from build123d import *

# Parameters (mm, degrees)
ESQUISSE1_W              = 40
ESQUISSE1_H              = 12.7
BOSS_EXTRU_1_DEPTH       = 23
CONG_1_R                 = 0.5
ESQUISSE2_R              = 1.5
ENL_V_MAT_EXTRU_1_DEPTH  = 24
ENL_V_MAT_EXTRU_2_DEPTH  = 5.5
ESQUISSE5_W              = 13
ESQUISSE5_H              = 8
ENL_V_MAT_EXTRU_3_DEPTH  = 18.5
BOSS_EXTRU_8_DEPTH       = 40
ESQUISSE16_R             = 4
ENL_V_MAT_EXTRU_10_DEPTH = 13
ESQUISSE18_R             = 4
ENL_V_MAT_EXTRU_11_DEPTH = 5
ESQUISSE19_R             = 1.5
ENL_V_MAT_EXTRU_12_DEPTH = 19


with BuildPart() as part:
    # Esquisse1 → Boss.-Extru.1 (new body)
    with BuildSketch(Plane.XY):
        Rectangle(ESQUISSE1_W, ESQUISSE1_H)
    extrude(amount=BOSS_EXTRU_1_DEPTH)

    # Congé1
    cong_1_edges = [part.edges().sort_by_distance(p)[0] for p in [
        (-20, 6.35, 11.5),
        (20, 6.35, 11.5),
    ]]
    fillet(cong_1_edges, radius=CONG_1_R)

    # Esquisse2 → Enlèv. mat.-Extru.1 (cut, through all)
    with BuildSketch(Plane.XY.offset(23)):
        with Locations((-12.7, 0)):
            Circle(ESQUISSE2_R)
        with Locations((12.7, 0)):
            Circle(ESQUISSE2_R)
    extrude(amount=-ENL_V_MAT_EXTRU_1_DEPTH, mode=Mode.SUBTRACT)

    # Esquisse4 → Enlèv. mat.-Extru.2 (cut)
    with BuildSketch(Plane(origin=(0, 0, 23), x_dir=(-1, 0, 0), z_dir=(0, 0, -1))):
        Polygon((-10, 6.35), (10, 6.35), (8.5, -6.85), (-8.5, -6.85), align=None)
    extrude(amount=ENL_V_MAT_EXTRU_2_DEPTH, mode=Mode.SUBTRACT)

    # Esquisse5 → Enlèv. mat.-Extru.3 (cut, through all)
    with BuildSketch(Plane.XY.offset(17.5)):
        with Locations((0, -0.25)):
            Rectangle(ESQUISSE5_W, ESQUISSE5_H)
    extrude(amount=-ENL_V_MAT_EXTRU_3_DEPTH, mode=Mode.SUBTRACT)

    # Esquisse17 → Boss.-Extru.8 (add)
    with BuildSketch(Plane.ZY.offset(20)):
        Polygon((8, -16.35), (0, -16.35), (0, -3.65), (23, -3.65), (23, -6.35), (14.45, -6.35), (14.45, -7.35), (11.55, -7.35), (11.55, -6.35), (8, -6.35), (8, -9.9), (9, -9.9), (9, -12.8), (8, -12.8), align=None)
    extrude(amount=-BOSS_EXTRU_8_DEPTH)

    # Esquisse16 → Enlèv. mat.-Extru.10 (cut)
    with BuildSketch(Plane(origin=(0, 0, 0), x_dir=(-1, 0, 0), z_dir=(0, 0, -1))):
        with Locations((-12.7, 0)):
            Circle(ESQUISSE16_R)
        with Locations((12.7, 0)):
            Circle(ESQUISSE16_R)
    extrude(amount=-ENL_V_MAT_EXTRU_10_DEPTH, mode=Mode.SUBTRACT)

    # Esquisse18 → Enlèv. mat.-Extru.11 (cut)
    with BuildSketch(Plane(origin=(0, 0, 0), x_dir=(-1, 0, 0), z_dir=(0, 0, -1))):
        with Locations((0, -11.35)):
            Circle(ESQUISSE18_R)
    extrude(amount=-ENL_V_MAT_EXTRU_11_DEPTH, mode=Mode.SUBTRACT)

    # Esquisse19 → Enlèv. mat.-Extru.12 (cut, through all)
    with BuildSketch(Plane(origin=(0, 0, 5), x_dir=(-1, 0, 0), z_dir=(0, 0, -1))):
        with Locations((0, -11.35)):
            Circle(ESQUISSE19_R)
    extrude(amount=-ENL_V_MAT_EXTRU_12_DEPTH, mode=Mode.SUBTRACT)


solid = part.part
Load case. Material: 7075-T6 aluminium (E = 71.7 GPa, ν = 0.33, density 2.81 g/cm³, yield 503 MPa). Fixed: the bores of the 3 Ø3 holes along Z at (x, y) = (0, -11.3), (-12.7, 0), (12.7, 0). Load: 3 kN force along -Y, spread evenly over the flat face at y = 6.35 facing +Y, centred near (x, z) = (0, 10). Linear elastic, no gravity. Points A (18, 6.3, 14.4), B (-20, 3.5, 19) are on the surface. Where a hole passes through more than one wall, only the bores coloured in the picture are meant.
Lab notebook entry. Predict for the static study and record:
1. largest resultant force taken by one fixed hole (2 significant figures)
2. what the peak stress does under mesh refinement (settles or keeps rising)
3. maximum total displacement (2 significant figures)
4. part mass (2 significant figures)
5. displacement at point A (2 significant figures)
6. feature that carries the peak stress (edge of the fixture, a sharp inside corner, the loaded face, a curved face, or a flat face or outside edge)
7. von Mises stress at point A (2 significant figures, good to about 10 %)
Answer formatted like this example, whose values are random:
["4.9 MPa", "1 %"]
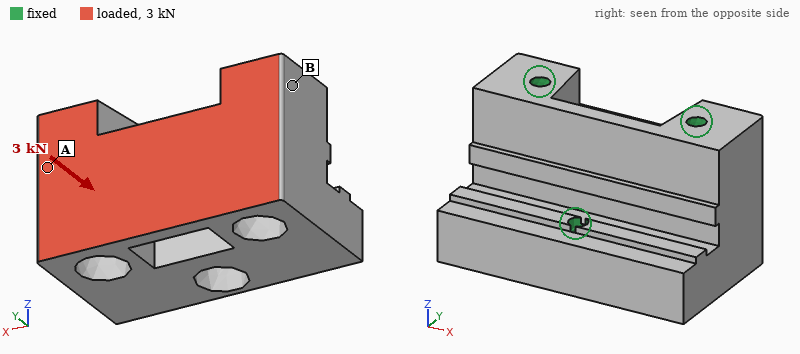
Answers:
["1.1 kN", "keeps rising", "15 µm", "30 g", "2.5 µm", "edge of the fixture", "11 MPa"]
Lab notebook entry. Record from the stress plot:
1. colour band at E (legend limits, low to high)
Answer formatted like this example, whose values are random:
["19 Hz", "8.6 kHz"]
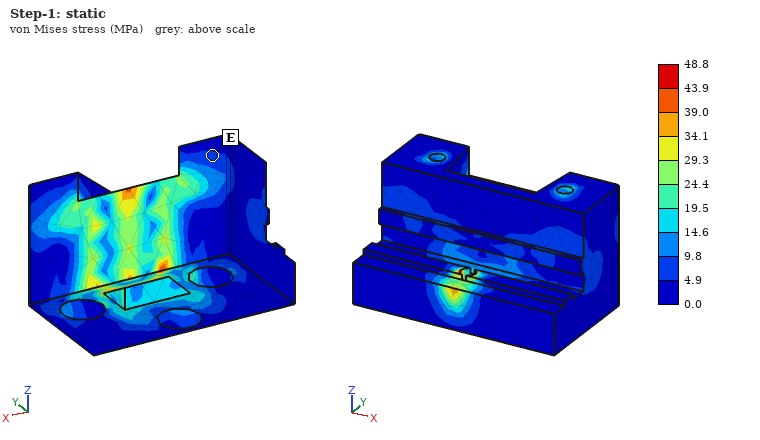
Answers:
["4.9 to 9.8 MPa"]
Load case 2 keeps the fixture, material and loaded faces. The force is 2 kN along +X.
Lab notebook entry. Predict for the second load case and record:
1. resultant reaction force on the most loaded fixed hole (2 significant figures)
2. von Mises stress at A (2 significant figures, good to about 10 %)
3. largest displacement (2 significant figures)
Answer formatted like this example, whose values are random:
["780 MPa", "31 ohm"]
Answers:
["1.1 kN", "7.5 MPa", "9.4 µm"]
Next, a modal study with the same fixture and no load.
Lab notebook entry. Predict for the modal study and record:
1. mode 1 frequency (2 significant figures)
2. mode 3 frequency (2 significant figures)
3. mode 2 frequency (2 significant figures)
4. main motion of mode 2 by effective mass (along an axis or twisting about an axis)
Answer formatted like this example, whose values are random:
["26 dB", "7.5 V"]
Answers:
["18 kHz", "28 kHz", "19 kHz", "along Y"]
